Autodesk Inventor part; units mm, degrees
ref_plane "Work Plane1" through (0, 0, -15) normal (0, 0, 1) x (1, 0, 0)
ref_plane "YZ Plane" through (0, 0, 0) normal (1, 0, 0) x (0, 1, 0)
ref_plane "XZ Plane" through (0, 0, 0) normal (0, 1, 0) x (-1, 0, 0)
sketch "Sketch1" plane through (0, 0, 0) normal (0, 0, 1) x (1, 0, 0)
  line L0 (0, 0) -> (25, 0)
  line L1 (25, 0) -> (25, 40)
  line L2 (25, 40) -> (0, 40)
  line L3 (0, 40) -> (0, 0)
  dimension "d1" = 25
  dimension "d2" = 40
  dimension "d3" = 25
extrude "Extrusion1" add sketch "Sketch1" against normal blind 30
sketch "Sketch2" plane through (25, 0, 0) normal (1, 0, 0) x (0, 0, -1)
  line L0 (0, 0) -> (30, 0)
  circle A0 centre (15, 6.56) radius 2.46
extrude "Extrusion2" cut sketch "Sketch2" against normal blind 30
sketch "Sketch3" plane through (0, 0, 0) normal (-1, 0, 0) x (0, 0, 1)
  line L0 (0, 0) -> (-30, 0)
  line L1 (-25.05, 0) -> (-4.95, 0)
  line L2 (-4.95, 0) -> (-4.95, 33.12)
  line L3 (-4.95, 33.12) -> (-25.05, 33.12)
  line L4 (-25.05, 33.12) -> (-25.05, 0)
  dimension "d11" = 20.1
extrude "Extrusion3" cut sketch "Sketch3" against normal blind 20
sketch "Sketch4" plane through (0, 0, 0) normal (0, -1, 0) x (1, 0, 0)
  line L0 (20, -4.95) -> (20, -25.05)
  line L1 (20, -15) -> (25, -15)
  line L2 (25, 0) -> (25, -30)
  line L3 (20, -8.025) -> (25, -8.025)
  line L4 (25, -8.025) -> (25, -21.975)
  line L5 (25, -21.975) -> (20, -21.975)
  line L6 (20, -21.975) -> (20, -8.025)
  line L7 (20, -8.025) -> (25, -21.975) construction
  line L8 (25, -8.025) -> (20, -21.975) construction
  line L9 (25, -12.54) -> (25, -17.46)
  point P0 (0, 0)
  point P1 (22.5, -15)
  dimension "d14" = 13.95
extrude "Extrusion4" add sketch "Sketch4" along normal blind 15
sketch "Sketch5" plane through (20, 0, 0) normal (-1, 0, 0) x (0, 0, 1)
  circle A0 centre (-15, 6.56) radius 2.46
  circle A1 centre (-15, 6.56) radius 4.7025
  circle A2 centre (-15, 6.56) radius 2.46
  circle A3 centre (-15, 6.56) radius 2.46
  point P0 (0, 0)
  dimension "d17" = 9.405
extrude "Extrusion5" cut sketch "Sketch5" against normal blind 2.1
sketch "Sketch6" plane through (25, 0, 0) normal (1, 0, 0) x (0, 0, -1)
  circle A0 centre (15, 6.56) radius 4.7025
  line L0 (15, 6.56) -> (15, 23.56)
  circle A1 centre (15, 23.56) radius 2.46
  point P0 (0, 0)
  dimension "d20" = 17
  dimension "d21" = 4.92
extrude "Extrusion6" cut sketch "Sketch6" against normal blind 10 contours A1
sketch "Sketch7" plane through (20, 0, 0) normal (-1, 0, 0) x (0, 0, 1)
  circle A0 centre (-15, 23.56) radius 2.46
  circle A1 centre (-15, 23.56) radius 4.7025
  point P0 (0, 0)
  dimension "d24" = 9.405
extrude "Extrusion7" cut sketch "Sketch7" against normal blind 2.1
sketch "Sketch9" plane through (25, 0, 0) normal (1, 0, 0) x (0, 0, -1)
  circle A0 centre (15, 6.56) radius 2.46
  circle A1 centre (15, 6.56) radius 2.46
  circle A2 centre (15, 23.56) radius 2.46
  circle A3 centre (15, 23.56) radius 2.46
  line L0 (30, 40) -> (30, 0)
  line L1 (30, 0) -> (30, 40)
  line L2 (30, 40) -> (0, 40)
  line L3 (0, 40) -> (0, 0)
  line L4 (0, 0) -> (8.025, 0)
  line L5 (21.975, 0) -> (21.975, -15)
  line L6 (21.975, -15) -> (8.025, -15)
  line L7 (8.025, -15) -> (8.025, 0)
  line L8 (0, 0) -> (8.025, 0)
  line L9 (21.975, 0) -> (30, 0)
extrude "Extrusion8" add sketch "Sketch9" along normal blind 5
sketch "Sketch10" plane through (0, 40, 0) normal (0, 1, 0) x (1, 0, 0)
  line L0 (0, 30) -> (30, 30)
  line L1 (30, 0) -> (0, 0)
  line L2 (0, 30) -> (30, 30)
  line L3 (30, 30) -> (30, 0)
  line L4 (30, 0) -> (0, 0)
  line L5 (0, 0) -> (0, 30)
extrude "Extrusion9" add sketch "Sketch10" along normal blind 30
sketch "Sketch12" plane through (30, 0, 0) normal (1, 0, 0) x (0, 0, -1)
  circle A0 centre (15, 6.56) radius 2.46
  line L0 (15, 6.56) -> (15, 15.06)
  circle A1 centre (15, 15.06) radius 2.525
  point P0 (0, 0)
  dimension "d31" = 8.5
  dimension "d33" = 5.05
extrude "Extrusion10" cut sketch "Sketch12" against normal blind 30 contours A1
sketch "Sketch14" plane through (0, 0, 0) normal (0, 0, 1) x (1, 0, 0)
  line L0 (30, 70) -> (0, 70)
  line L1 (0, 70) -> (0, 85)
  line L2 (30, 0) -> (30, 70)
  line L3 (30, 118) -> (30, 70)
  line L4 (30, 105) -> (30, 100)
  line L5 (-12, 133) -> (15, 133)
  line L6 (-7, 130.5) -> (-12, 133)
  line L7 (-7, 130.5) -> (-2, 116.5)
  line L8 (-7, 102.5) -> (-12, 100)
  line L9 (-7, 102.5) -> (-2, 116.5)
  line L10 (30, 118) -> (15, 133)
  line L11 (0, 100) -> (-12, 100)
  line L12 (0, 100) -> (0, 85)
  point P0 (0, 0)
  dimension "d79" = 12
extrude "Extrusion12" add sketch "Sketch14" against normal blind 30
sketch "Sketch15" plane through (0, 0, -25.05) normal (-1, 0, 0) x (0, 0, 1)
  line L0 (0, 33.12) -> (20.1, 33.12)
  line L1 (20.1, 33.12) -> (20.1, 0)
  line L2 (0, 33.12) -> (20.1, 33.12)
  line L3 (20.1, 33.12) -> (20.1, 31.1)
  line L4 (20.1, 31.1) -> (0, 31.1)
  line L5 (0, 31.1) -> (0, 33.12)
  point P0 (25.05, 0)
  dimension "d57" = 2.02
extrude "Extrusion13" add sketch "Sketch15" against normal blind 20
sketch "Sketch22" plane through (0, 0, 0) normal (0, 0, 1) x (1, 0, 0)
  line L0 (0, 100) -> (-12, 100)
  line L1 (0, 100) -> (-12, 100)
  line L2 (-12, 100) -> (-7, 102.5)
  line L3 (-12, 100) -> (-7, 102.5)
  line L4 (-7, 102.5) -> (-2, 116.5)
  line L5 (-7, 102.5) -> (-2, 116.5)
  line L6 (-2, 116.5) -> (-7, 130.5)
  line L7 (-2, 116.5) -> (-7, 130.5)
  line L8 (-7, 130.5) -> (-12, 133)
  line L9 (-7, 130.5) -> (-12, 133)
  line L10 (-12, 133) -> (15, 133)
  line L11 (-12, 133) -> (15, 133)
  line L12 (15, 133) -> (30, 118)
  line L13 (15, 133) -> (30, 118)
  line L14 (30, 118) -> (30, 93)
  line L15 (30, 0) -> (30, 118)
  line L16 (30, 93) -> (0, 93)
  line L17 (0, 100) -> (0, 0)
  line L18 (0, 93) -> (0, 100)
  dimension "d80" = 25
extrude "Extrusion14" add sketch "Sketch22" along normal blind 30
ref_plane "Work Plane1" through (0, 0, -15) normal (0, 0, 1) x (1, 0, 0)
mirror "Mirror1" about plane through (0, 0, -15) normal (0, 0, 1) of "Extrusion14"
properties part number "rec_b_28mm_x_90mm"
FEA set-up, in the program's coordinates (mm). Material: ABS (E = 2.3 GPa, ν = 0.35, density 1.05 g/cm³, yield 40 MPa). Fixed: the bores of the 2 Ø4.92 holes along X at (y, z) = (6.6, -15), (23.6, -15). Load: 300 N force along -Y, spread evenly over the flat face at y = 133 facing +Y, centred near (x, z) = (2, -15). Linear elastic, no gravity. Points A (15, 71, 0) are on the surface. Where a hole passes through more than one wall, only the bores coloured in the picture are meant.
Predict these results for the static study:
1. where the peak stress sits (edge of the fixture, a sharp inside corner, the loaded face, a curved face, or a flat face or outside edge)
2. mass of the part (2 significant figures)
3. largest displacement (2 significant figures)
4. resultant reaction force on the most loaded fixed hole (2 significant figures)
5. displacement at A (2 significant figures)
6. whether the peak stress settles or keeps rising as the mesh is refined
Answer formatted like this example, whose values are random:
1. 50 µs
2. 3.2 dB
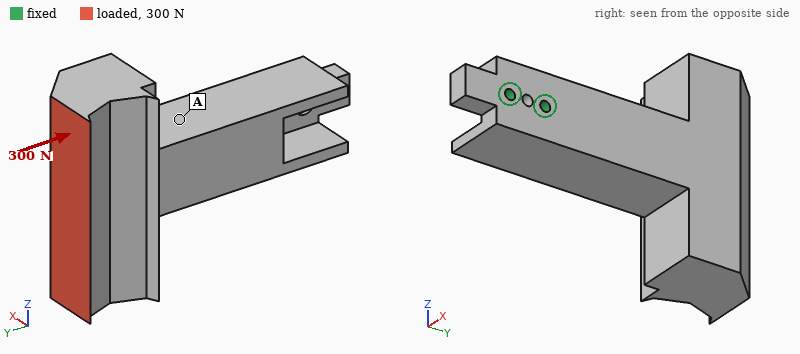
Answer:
1. edge of the fixture
2. 200 g
3. 0.70 mm
4. 340 N
5. 0.25 mm
6. keeps rising
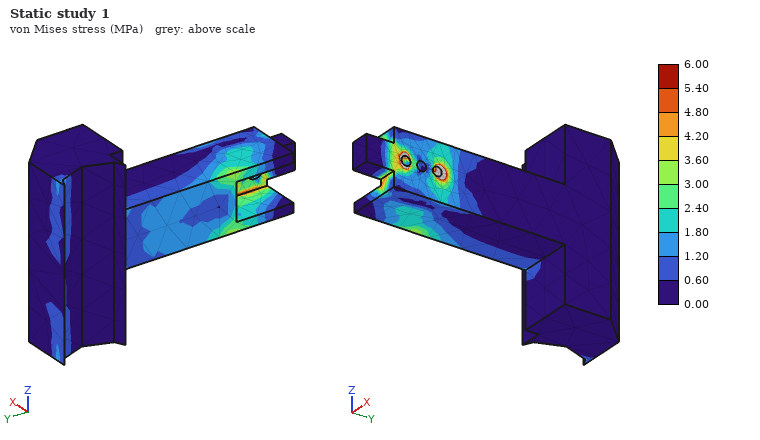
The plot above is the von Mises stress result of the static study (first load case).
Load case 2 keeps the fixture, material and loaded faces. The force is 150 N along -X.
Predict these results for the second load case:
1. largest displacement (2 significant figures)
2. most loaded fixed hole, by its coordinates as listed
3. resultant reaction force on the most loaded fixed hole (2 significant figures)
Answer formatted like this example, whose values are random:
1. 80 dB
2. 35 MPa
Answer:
1. 1.7 mm
2. (23.6, -15)
3. 810 N
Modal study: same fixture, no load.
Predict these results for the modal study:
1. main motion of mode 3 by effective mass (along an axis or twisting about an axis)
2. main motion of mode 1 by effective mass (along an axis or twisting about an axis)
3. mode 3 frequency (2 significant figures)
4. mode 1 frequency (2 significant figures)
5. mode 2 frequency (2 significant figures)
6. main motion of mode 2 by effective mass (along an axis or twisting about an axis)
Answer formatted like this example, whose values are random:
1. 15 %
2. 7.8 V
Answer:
1. twisting about Y
2. along X
3. 350 Hz
4. 170 Hz
5. 190 Hz
6. along Z
